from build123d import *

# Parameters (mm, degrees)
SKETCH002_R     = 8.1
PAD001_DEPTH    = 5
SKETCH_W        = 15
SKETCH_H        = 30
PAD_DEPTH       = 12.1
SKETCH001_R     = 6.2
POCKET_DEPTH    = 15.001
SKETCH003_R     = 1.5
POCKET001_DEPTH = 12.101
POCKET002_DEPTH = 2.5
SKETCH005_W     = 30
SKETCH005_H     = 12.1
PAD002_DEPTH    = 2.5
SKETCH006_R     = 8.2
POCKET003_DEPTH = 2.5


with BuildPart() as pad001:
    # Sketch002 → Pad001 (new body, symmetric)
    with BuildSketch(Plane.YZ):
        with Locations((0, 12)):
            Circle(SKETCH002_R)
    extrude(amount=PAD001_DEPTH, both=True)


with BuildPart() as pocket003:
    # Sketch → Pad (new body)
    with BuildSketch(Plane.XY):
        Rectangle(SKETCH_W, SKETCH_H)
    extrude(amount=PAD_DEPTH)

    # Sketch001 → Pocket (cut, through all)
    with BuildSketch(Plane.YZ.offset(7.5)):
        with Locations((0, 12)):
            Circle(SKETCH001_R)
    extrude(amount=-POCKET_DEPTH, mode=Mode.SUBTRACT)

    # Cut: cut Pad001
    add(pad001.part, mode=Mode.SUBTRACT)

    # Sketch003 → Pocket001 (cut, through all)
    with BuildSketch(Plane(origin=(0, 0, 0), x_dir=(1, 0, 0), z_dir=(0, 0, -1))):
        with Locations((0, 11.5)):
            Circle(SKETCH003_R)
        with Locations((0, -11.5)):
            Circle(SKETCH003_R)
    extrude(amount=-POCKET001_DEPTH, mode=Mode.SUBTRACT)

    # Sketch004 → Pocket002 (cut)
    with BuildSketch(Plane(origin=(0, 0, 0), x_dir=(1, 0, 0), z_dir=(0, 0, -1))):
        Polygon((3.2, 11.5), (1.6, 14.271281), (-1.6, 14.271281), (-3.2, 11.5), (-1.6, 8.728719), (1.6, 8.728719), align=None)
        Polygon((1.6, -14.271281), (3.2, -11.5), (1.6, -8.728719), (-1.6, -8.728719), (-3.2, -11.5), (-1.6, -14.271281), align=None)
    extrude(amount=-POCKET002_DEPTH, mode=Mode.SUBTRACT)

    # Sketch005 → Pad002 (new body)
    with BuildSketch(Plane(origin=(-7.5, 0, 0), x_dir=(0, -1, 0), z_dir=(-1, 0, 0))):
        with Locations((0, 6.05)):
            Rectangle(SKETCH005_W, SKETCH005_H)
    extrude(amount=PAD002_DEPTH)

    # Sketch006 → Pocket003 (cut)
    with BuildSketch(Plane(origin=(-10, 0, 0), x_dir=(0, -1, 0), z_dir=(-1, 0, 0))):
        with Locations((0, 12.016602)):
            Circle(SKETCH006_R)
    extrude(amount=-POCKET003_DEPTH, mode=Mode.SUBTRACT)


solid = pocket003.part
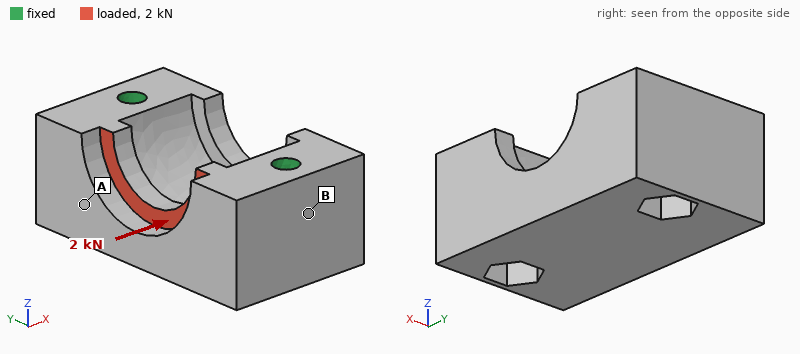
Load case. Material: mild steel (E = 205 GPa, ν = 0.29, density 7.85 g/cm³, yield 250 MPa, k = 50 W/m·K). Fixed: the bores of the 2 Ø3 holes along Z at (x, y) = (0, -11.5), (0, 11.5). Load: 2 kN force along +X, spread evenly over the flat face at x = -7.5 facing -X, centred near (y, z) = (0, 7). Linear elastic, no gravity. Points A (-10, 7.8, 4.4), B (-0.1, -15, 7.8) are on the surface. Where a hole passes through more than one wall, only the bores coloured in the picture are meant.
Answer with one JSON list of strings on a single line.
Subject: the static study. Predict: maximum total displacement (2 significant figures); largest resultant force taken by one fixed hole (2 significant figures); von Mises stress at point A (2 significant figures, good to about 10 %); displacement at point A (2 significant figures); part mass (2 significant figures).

["3.5 µm", "1.0 kN", "17 MPa", "1.4 µm", "35 g"]
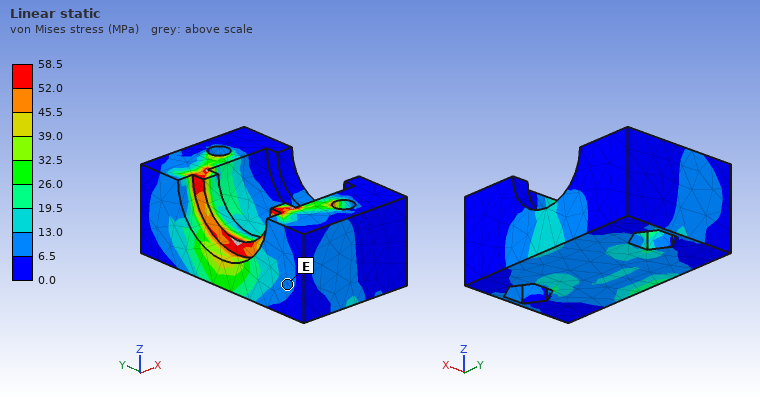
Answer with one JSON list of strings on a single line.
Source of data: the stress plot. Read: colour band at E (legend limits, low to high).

["6.5 to 13.0 MPa"]
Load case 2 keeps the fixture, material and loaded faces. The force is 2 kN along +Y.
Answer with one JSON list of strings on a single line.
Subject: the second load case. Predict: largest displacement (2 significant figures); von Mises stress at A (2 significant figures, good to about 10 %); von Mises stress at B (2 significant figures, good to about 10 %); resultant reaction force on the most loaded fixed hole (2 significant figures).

["3.7 µm", "9.6 MPa", "18 MPa", "1.1 kN"]
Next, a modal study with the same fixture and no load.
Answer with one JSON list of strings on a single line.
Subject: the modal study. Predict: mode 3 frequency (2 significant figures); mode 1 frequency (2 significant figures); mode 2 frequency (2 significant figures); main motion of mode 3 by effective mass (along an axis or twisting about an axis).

["48 kHz", "35 kHz", "46 kHz", "along Z"]
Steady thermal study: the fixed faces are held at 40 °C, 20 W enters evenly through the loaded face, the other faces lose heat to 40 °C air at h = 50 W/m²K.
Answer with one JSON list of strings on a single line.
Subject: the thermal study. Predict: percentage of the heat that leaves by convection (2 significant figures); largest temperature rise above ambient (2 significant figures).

["4.1 %", "35 K"]
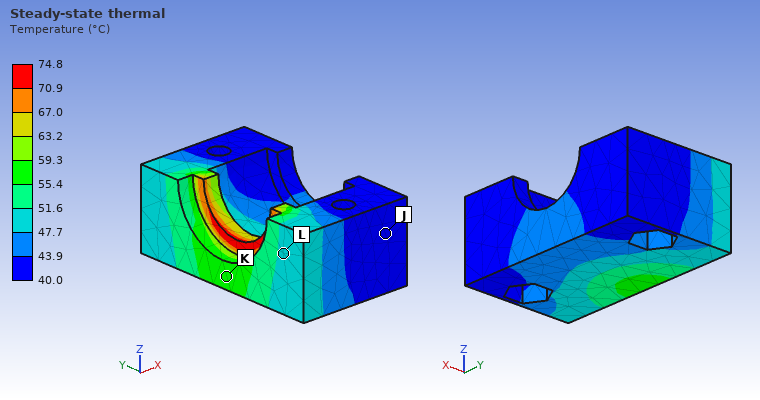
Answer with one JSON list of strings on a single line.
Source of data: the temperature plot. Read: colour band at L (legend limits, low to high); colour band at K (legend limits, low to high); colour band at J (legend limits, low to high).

["47.7 to 51.6 °C", "55.4 to 59.3 °C", "40.0 to 43.9 °C"]
